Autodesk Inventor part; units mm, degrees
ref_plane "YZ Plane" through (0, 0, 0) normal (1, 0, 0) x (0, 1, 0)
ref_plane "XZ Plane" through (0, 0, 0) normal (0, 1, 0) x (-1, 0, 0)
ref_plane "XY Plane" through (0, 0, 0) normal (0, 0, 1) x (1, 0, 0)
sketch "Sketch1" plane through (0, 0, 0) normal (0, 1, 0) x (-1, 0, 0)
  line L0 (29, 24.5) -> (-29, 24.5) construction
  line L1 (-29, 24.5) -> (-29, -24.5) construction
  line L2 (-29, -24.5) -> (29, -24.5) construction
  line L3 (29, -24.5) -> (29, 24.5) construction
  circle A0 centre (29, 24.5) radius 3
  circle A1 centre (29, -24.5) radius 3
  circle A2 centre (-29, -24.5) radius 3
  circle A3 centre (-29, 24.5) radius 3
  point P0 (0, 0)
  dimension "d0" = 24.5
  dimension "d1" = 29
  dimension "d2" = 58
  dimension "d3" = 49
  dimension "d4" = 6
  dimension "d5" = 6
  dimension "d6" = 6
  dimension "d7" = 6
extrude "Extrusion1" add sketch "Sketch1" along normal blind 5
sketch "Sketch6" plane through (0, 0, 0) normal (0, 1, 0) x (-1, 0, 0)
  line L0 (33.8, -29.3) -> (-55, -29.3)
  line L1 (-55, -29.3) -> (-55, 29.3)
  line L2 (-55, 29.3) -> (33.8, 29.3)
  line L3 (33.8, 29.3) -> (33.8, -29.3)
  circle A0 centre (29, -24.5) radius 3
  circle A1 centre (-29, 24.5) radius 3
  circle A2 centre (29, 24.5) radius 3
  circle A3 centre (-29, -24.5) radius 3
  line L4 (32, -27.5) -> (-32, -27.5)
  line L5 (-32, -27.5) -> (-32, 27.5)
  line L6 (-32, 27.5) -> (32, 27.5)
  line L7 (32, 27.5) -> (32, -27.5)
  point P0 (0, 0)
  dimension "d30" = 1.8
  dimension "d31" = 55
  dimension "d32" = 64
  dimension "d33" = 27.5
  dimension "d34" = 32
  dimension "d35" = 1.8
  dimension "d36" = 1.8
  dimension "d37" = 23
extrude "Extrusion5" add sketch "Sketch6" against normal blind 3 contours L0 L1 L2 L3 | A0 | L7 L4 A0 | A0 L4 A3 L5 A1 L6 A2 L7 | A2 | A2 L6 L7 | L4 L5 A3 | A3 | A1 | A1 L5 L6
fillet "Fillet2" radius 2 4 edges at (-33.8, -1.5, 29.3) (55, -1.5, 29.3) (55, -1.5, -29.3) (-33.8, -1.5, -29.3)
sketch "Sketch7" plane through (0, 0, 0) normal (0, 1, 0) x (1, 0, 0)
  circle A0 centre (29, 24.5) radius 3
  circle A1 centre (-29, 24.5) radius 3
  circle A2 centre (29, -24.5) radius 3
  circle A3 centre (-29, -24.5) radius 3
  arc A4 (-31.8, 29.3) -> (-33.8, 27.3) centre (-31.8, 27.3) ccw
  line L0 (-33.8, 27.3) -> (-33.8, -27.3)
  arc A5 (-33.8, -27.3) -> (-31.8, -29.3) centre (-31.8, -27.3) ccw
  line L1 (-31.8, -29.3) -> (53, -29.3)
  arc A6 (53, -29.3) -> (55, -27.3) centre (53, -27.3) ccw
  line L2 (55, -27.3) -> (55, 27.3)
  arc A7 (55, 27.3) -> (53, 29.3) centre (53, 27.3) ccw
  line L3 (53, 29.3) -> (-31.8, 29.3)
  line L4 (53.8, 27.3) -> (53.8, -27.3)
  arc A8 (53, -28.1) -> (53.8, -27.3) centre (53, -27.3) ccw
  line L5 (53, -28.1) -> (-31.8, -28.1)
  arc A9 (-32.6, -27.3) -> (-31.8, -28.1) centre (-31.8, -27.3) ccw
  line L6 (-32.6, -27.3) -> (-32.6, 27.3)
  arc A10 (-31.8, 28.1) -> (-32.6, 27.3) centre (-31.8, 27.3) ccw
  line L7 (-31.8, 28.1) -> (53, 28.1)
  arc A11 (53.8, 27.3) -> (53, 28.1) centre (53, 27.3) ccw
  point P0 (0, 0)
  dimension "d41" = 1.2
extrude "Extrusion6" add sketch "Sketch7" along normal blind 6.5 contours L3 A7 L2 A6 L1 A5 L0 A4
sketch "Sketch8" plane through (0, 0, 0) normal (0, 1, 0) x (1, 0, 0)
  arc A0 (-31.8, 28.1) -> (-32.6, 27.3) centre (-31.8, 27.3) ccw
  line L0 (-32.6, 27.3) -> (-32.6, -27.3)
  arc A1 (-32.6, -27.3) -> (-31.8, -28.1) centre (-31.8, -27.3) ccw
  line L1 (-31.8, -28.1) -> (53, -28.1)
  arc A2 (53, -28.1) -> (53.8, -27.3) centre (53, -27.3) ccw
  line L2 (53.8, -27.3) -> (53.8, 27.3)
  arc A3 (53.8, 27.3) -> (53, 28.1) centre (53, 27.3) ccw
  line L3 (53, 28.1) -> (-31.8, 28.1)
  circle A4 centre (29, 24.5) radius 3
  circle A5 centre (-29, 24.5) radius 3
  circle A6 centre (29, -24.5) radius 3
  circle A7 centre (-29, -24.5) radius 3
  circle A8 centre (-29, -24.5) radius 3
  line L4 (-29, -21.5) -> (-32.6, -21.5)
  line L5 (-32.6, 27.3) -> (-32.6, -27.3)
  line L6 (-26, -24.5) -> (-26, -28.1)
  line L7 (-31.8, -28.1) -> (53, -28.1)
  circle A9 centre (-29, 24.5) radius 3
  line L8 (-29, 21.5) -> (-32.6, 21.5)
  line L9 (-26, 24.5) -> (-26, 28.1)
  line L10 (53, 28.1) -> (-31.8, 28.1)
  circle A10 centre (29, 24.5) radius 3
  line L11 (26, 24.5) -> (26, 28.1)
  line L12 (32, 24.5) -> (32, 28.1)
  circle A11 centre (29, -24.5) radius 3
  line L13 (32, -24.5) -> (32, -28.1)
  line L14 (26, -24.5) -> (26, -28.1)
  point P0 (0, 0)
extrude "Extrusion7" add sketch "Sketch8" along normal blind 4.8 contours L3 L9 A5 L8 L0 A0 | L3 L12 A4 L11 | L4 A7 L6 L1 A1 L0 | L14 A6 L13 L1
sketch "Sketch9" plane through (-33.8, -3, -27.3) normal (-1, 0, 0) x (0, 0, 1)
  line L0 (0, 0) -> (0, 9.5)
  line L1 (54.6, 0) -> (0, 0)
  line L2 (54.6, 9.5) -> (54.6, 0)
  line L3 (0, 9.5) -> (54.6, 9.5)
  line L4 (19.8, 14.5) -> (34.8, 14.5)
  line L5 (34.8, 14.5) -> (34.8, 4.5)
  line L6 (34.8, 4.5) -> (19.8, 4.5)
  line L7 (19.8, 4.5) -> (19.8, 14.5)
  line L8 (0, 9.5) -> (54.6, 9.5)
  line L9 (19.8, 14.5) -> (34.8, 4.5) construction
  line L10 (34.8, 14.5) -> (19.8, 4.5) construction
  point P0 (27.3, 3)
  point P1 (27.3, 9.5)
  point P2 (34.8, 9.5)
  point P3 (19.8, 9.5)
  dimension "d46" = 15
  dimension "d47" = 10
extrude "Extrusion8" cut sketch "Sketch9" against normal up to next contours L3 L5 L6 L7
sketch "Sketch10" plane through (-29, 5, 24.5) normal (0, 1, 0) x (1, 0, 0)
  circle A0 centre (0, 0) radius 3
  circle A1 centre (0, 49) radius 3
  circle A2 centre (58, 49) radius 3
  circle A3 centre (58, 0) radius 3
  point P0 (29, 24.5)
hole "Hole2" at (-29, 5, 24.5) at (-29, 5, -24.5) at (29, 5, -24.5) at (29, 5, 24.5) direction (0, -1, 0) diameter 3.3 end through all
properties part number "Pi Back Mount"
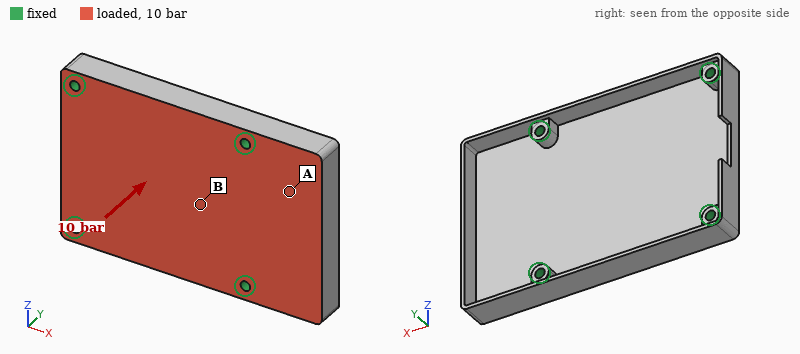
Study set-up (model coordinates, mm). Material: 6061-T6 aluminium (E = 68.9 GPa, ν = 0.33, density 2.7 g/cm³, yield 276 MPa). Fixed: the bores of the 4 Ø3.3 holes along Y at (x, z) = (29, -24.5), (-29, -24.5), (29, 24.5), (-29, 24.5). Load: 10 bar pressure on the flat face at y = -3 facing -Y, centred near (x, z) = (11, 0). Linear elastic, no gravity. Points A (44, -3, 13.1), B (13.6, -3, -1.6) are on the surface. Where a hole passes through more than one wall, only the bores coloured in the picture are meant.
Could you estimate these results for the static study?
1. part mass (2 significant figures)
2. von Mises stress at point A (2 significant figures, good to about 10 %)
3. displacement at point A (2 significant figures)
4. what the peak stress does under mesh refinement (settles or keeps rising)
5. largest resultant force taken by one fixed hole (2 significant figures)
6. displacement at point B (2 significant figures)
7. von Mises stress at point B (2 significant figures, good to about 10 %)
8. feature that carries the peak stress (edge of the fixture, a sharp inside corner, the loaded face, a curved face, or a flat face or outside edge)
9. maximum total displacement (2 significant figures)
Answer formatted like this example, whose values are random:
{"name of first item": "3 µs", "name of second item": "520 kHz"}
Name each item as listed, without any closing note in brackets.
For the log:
{"part mass": "49 g", "von Mises stress at point A": "35 MPa", "displacement at point A": "0.13 mm", "what the peak stress does under mesh refinement": "keeps rising", "largest resultant force taken by one fixed hole": "1.7 kN", "displacement at point B": "0.22 mm", "von Mises stress at point B": "81 MPa", "feature that carries the peak stress": "edge of the fixture", "maximum total displacement": "0.26 mm"}
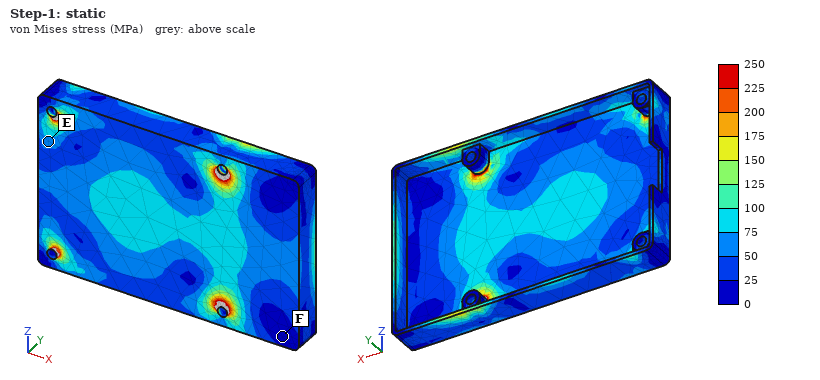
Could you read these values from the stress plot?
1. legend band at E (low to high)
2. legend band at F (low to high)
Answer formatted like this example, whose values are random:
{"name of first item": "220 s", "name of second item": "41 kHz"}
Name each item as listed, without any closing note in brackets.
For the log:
{"legend band at E": "50 to 75 MPa", "legend band at F": "0 to 25 MPa"}
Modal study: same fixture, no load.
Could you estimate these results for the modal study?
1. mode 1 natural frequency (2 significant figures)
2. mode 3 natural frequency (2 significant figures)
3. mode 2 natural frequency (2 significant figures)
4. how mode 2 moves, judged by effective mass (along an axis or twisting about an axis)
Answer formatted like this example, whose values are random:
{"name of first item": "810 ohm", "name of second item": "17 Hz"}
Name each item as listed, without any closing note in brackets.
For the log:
{"mode 1 natural frequency": "3900 Hz", "mode 3 natural frequency": "7000 Hz", "mode 2 natural frequency": "4300 Hz", "how mode 2 moves, judged by effective mass": "along Y"}
